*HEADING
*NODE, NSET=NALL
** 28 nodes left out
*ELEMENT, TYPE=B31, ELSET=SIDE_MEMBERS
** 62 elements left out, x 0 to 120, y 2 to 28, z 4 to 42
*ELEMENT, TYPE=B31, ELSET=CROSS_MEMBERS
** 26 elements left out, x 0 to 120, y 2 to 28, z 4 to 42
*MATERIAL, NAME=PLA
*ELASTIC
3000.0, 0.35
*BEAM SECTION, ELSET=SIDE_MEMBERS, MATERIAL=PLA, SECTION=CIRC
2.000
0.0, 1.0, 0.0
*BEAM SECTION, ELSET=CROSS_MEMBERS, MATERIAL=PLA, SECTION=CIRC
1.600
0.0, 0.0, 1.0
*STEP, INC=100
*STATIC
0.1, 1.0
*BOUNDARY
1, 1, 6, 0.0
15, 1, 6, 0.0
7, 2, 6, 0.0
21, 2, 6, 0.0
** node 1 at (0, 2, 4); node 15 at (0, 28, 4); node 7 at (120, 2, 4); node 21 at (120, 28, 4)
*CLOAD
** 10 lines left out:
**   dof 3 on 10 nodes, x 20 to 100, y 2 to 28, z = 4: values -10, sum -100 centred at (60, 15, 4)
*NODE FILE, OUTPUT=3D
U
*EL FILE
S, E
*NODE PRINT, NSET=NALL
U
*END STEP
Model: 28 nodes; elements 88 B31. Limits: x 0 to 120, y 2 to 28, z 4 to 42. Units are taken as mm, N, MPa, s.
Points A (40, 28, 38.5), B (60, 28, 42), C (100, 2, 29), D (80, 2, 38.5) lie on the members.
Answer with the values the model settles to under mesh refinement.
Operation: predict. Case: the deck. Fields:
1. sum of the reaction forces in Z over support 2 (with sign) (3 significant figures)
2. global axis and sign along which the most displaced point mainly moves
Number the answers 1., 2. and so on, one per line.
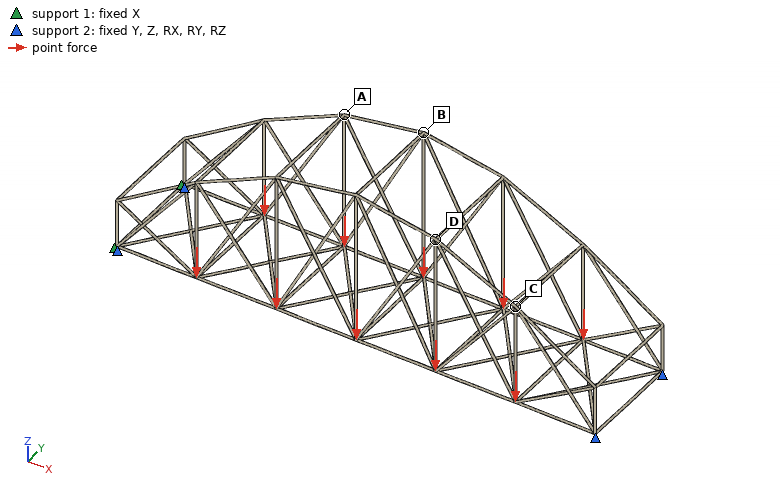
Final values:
1. 100 N
2. -Z
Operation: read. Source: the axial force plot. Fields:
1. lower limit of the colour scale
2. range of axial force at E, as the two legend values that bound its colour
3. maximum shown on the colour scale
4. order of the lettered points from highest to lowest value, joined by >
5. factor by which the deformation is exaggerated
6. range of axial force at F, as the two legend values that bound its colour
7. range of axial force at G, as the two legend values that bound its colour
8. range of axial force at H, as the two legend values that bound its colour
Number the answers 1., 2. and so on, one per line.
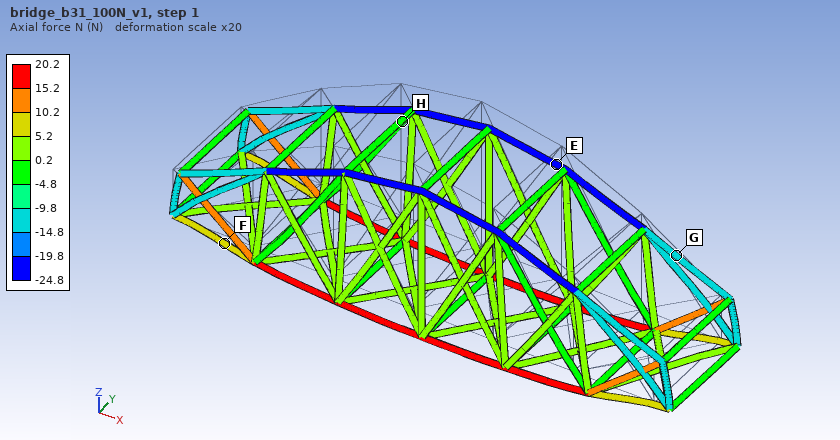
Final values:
1. -24.8 N
2. -24.8 to -19.8 N
3. 20.2 N
4. F > H > G > E
5. 20
6. 5.2 to 10.2 N
7. -14.8 to -9.8 N
8. -4.8 to 0.2 N
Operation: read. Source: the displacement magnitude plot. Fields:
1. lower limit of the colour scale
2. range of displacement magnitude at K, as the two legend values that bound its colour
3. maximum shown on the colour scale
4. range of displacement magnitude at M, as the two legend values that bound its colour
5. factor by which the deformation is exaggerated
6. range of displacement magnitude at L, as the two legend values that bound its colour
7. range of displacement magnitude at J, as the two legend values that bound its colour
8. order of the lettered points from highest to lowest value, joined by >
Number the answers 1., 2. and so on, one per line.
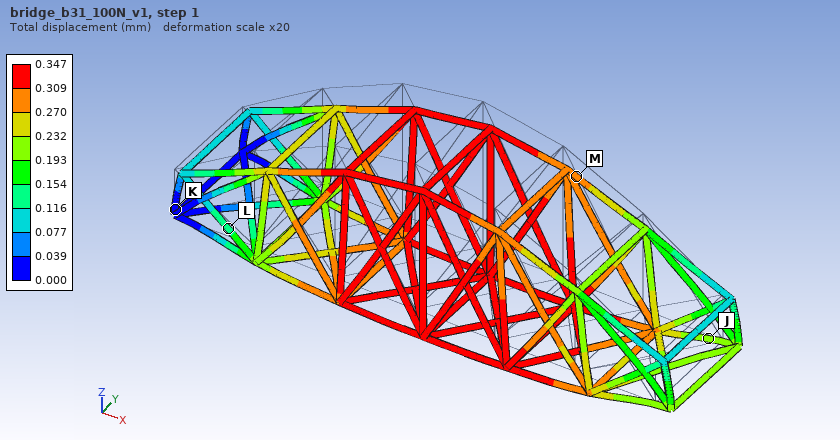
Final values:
1. 0.000 mm
2. 0.000 to 0.039 mm
3. 0.347 mm
4. 0.270 to 0.309 mm
5. 20
6. 0.116 to 0.154 mm
7. 0.193 to 0.232 mm
8. M > J > L > K
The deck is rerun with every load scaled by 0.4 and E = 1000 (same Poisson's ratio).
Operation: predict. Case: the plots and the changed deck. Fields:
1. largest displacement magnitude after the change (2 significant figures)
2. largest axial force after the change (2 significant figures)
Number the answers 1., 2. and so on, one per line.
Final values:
1. 0.42 mm
2. 8.1 N
